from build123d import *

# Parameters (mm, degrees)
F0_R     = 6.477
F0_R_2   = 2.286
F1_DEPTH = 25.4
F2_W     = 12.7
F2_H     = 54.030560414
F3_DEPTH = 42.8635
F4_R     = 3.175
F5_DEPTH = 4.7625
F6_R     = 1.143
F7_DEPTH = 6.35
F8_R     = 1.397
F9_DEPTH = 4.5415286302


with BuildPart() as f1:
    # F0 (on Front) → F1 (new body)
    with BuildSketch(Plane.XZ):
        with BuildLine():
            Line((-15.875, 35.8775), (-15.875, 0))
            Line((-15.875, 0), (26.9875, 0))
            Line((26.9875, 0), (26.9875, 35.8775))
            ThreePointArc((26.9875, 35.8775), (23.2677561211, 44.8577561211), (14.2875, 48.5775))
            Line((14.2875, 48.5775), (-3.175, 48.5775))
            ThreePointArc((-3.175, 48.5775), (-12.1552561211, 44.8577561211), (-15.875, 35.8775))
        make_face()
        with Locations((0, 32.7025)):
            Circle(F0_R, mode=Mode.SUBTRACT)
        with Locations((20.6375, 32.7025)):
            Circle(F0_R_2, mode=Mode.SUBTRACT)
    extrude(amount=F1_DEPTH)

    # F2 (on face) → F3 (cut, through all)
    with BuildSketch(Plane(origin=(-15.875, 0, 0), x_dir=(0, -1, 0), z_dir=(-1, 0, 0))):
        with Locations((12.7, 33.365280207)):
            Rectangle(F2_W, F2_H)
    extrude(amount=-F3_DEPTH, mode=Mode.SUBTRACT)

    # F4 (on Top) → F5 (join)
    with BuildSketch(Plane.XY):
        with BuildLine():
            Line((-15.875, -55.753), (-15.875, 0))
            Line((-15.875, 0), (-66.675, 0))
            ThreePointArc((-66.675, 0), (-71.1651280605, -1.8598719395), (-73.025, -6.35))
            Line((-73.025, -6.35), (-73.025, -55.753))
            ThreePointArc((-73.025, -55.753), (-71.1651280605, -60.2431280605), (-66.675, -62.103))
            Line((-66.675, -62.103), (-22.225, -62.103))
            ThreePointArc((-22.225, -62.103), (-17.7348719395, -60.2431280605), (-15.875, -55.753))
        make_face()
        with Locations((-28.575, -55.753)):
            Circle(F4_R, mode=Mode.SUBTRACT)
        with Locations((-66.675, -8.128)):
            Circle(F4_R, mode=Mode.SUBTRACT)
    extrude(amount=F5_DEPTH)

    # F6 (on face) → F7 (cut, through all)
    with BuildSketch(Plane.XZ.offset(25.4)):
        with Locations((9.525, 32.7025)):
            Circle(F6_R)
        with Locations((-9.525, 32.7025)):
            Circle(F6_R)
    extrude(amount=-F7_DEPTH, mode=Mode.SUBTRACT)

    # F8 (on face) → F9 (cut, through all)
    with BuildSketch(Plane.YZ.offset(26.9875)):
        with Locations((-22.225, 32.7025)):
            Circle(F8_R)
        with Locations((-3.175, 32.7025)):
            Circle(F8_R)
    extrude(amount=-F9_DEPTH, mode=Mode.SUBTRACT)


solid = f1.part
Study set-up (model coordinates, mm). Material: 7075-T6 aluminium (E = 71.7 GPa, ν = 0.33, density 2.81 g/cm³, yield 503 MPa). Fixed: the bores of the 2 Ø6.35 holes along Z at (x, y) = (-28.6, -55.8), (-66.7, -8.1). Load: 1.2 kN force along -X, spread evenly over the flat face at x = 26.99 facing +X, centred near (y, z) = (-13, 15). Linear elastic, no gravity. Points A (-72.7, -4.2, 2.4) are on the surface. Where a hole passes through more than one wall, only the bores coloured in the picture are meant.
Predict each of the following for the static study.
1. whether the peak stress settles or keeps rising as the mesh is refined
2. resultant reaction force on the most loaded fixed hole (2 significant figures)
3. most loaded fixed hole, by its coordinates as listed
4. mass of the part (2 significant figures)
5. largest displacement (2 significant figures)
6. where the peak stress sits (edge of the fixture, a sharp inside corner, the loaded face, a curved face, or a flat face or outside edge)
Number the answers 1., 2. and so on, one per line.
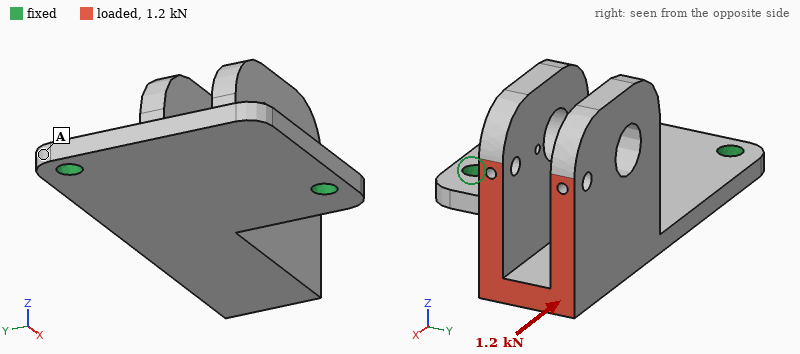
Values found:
1. keeps rising
2. 990 N
3. (-66.7, -8.1)
4. 120 g
5. 1.5 mm
6. a sharp inside corner
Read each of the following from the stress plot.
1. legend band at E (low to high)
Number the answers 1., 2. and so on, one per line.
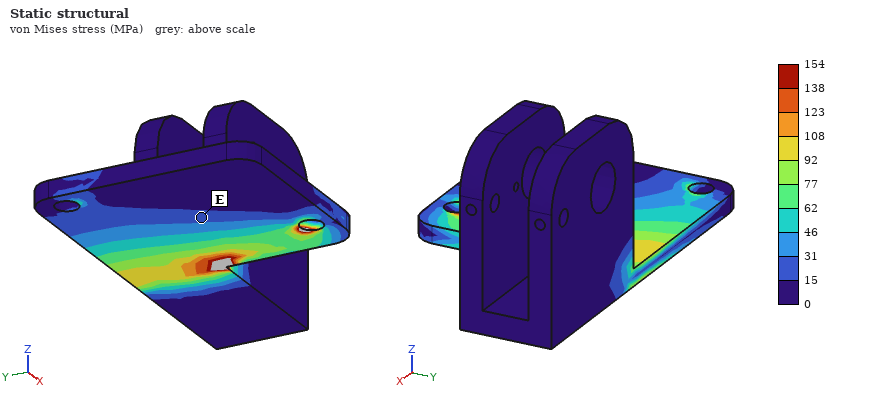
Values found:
1. 15 to 31 MPa
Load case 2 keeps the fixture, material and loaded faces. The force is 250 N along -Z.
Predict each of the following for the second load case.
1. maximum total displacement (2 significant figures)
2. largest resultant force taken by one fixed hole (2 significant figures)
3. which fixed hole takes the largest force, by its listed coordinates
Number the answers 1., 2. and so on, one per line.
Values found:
1. 1.5 mm
2. 290 N
3. (-28.6, -55.8)
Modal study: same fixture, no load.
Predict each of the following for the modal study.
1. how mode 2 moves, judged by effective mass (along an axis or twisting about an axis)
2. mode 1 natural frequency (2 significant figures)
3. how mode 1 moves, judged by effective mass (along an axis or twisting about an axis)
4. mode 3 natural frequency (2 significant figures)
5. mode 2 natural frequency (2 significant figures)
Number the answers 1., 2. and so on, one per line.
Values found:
1. along Y
2. 330 Hz
3. along Z
4. 1800 Hz
5. 790 Hz
